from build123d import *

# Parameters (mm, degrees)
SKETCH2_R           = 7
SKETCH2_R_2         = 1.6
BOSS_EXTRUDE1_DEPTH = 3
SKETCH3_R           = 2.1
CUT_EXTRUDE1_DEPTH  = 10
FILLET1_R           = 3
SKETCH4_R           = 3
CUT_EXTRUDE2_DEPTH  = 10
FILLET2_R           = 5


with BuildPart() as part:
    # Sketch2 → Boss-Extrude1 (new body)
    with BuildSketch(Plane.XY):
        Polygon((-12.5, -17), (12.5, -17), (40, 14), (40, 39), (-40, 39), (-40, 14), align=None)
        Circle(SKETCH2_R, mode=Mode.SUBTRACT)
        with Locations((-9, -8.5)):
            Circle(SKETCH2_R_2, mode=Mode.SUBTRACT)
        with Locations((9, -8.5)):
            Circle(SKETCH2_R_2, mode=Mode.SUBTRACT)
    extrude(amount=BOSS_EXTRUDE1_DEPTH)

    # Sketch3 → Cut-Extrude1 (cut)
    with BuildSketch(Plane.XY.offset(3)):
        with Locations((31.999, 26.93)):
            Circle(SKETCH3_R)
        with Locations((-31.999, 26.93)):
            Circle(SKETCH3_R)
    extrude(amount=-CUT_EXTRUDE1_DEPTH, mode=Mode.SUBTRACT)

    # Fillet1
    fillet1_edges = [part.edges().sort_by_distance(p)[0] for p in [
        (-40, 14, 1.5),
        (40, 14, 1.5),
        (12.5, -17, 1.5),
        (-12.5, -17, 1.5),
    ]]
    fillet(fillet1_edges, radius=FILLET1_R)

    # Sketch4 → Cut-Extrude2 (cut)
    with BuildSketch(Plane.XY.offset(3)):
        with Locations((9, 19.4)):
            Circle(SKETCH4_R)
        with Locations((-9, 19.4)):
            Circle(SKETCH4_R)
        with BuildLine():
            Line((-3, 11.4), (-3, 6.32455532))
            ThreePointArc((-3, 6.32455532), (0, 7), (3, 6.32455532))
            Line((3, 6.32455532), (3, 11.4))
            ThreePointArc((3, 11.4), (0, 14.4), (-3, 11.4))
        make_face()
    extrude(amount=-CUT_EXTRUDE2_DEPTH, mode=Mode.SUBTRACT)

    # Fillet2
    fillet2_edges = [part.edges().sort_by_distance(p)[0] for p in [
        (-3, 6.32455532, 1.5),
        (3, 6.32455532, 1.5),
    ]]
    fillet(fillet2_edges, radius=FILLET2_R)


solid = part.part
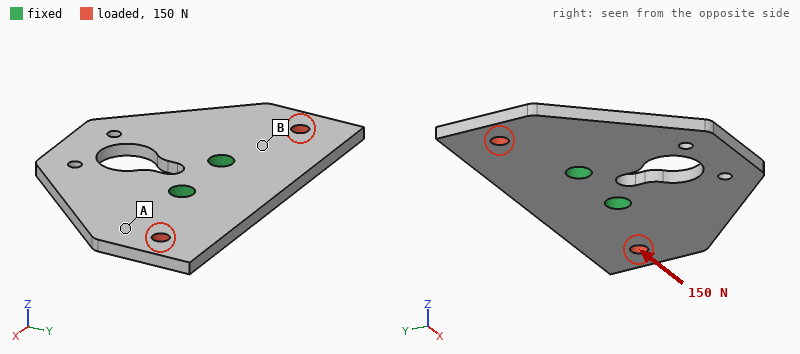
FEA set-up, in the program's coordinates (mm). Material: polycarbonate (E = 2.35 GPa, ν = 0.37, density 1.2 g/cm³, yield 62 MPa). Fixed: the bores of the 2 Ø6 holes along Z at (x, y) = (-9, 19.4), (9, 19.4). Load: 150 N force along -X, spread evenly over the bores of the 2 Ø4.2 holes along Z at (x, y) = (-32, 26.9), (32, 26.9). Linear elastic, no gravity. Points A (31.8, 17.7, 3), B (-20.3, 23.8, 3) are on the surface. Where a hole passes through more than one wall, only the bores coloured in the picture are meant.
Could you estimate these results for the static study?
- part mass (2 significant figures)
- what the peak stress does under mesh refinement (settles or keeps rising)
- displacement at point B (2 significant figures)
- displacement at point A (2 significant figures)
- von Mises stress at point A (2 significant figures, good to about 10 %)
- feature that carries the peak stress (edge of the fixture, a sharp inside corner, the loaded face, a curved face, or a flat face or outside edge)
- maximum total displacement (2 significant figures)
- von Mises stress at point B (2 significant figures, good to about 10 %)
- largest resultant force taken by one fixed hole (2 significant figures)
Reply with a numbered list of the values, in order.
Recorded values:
1. 12 g
2. keeps rising
3. 14 µm
4. 21 µm
5. 0.51 MPa
6. edge of the fixture
7. 36 µm
8. 1.5 MPa
9. 86 N
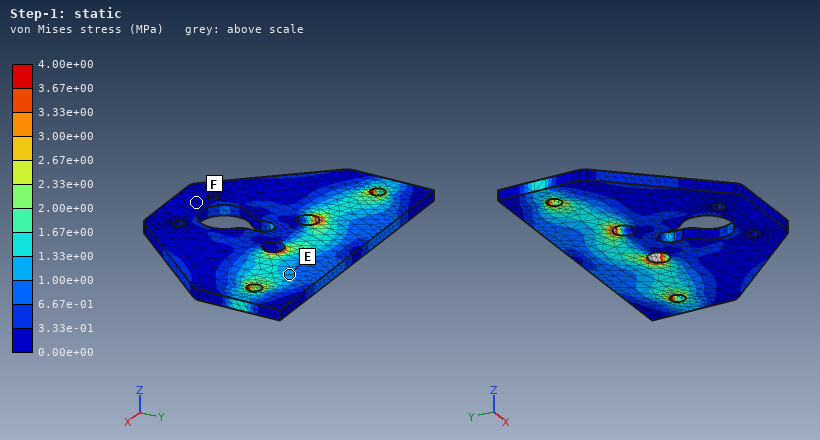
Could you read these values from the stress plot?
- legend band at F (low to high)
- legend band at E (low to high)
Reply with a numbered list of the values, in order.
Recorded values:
1. 0.00e+00 to 3.33e-01 MPa
2. 1.00e+00 to 1.33e+00 MPa
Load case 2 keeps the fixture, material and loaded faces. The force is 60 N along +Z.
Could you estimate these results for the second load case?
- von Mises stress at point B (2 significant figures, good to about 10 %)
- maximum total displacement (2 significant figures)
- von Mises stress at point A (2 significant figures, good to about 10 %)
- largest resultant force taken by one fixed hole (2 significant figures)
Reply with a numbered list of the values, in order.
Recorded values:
1. 6.4 MPa
2. 1.2 mm
3. 3.1 MPa
4. 30 N
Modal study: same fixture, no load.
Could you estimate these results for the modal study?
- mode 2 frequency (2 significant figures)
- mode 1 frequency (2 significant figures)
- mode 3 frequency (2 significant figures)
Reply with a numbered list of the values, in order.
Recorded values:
1. 800 Hz
2. 630 Hz
3. 800 Hz
